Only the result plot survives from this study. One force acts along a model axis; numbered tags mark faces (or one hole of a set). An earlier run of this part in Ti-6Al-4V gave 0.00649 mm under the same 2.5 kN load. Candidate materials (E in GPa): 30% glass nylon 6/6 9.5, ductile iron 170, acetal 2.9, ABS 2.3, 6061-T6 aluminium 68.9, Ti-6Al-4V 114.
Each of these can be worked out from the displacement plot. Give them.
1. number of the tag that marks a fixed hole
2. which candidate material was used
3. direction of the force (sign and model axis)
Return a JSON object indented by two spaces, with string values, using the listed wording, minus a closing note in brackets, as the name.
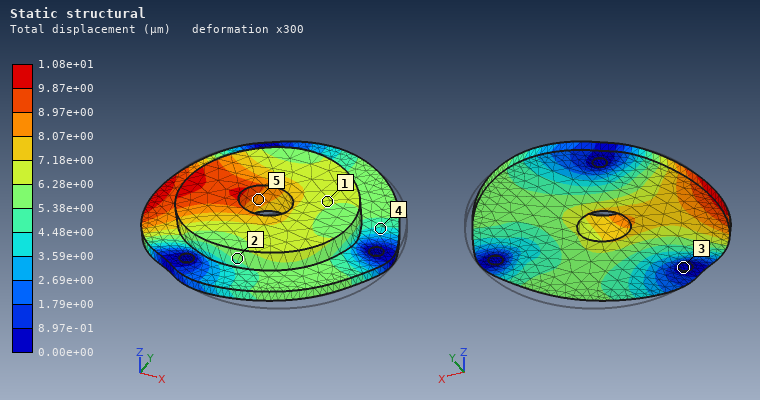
{
  "number of the tag that marks a fixed hole": "3",
  "which candidate material was used": "6061-T6 aluminium",
  "direction of the force": "-X"
}
